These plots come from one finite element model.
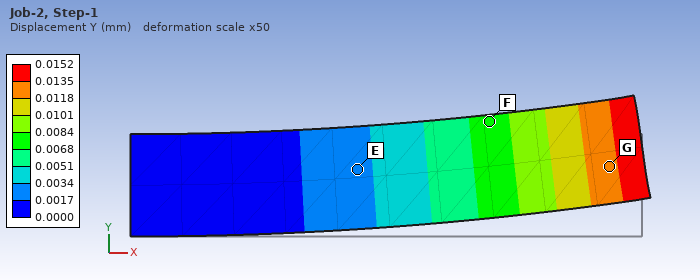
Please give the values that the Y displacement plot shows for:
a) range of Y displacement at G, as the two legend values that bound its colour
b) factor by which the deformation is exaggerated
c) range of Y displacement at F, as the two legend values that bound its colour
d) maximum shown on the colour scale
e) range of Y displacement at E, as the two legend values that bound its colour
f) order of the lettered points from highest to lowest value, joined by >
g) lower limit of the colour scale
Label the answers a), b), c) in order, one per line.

a) 0.0118 to 0.0135 mm
b) 50
c) 0.0068 to 0.0084 mm
d) 0.0152 mm
e) 0.0017 to 0.0034 mm
f) G > F > E
g) 0.0000 mm
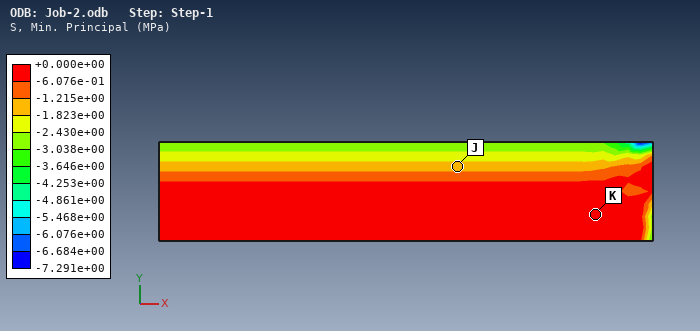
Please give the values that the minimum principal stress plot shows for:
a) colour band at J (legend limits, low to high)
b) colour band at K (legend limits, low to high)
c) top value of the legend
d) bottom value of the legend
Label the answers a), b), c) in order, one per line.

a) -1.823e+00 to -1.215e+00 MPa
b) -6.076e-01 to +0.000e+00 MPa
c) +0.000e+00 MPa
d) -7.291e+00 MPa
